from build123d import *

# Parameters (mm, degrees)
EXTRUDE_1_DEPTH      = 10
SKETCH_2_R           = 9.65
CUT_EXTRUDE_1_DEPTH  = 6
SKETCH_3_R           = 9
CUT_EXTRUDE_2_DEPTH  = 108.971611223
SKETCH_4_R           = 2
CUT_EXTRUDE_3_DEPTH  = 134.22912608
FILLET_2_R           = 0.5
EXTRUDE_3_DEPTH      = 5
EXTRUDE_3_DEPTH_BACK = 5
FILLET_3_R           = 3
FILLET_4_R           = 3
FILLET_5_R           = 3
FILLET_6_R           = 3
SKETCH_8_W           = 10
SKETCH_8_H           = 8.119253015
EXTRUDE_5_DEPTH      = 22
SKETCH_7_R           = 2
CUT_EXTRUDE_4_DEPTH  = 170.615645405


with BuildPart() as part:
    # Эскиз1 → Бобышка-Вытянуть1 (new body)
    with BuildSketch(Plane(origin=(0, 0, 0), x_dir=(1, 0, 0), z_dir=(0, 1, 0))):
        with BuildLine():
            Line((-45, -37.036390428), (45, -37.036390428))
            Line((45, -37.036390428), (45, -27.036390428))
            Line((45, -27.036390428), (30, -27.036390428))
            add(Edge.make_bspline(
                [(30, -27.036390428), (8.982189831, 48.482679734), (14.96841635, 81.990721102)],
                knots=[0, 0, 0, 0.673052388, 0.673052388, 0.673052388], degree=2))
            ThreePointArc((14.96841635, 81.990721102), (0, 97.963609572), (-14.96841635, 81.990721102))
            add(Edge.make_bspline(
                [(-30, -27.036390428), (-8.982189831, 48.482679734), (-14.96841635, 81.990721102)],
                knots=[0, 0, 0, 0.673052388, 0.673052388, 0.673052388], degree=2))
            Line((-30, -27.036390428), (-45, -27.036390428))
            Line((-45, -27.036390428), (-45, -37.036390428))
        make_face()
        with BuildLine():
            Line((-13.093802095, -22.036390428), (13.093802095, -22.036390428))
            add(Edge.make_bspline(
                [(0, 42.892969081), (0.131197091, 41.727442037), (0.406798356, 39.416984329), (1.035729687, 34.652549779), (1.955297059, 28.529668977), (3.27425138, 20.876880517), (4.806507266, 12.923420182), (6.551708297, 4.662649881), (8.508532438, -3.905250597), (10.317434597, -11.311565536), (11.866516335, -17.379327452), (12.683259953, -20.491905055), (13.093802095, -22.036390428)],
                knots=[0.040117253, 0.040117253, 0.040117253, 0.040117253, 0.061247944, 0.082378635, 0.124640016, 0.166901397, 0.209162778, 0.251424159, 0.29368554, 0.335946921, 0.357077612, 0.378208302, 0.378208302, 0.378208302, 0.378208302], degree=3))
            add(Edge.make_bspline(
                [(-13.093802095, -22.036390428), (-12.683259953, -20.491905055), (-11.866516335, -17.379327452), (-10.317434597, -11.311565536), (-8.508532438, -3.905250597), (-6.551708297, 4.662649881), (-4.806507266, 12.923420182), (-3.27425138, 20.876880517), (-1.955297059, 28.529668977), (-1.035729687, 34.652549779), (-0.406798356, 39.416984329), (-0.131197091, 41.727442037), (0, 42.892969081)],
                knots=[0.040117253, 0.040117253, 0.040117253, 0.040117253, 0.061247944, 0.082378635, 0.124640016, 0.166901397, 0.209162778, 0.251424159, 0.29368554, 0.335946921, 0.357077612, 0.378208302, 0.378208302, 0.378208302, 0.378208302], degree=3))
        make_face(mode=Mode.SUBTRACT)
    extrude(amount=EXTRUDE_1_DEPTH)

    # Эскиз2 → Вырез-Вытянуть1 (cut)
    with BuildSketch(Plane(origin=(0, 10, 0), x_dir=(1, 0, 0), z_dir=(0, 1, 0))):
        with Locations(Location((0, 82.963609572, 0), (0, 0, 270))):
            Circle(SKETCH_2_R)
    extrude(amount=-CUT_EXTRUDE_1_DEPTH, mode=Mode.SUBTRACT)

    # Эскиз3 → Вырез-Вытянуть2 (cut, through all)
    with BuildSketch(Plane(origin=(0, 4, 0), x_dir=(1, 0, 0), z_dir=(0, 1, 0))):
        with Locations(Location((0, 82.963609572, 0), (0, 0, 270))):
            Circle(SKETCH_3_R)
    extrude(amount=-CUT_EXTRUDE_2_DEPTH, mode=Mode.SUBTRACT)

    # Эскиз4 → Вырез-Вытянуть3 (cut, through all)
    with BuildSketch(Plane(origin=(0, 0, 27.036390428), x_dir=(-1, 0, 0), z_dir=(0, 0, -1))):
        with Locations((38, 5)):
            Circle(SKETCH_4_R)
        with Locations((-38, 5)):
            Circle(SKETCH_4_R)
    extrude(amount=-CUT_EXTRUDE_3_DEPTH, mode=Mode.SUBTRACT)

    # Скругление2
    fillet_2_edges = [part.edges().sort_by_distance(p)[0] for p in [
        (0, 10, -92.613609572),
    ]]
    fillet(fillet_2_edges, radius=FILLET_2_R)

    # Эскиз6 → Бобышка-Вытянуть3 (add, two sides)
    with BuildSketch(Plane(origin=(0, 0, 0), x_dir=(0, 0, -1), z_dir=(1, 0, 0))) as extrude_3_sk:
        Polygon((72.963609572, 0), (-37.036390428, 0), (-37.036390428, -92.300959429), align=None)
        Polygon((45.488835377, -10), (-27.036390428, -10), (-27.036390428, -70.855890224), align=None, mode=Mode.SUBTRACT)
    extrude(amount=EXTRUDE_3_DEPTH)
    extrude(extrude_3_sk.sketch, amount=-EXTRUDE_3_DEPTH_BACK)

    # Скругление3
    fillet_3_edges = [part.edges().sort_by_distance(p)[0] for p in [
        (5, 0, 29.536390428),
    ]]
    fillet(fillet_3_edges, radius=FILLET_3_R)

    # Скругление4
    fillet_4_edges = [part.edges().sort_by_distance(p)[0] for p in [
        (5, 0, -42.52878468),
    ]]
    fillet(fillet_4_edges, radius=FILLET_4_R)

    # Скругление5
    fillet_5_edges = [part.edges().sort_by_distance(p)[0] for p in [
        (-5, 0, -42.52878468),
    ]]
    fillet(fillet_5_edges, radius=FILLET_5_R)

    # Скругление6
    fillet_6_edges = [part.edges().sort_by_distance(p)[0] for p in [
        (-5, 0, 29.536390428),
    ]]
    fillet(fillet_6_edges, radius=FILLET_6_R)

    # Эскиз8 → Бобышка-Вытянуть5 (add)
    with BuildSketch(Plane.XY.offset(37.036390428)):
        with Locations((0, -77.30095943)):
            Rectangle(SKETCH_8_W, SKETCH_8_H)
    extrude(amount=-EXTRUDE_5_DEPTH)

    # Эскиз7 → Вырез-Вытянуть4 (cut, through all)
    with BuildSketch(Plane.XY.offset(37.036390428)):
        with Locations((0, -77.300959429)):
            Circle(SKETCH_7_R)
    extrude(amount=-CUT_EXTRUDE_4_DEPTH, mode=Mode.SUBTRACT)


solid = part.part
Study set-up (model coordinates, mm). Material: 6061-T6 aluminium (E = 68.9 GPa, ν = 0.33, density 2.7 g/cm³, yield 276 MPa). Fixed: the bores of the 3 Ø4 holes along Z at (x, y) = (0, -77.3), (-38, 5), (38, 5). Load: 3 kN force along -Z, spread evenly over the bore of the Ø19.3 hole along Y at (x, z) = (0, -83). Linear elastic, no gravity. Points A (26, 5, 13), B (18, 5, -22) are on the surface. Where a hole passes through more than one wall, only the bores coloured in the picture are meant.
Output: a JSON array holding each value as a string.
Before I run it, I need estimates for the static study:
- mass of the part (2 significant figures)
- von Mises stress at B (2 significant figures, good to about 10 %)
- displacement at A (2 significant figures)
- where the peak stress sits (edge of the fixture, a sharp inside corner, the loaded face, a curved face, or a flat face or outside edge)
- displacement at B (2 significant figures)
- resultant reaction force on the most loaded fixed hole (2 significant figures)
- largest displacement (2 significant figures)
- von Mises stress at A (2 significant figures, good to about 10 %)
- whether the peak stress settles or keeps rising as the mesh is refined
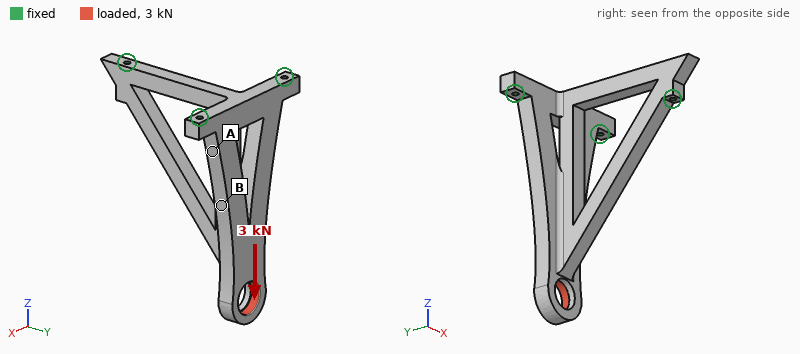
["200 g", "9.3 MPa", "0.016 mm", "edge of the fixture", "0.024 mm", "1.7 kN", "0.10 mm", "20 MPa", "keeps rising"]
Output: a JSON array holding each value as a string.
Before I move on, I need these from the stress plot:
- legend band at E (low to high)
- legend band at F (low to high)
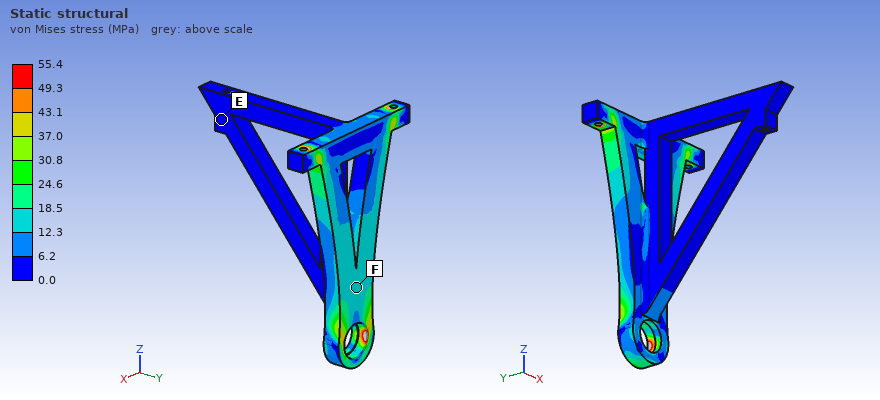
["0.0 to 6.2 MPa", "12.3 to 18.5 MPa"]
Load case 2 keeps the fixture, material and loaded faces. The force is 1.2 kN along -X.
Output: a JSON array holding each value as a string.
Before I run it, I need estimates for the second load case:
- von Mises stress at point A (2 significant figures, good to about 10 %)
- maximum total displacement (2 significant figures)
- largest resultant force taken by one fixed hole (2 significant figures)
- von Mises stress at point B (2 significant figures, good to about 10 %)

["32 MPa", "0.26 mm", "2.2 kN", "34 MPa"]
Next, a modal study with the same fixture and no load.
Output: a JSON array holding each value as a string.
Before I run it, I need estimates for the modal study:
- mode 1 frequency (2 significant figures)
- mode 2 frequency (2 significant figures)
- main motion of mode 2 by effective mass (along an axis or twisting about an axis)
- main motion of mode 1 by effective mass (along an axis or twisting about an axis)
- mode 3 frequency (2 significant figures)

["2200 Hz", "2700 Hz", "along Y", "along X", "3200 Hz"]
